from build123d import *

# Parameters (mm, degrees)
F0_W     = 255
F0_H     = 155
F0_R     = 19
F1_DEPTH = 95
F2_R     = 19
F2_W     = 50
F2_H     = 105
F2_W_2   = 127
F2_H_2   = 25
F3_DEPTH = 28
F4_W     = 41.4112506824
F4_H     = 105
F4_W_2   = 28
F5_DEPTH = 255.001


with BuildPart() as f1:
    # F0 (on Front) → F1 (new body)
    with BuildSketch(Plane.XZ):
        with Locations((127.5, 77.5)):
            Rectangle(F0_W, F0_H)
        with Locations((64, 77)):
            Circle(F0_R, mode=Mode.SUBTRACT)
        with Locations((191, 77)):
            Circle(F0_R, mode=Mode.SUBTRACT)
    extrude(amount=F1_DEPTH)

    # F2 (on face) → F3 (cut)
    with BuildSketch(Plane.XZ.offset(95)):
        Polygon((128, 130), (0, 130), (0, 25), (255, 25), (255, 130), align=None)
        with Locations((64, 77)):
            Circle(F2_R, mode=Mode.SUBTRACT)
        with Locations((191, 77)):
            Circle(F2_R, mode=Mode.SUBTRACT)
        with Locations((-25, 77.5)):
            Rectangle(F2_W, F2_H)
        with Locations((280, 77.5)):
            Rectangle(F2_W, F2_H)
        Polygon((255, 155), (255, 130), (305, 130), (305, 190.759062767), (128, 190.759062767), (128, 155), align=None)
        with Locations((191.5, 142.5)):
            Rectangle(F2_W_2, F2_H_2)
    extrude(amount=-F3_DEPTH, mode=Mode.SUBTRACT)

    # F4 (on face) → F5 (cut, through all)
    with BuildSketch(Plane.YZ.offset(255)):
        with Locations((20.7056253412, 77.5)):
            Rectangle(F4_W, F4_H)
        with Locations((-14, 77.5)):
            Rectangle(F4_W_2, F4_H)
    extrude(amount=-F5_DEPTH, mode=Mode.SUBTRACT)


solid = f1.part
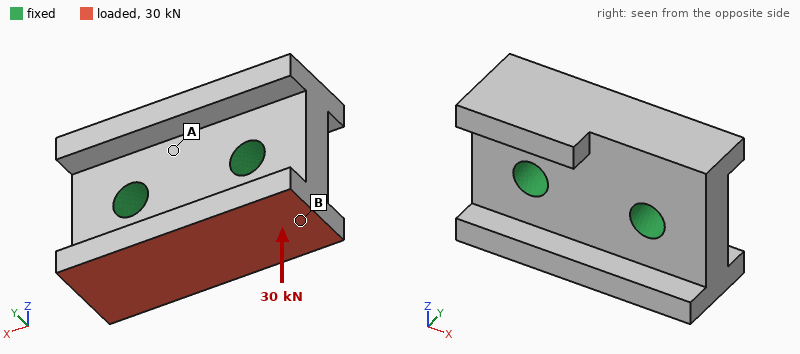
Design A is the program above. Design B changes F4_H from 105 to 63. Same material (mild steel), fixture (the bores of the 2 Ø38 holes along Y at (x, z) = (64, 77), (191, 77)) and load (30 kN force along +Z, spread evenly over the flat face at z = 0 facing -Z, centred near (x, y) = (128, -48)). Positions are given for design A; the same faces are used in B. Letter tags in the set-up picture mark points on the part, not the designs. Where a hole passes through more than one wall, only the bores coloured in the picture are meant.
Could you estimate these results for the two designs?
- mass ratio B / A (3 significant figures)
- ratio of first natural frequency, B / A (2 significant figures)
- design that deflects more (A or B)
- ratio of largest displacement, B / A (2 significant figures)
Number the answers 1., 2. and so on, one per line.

1. 1.14
2. 0.97
3. B
4. 1.1
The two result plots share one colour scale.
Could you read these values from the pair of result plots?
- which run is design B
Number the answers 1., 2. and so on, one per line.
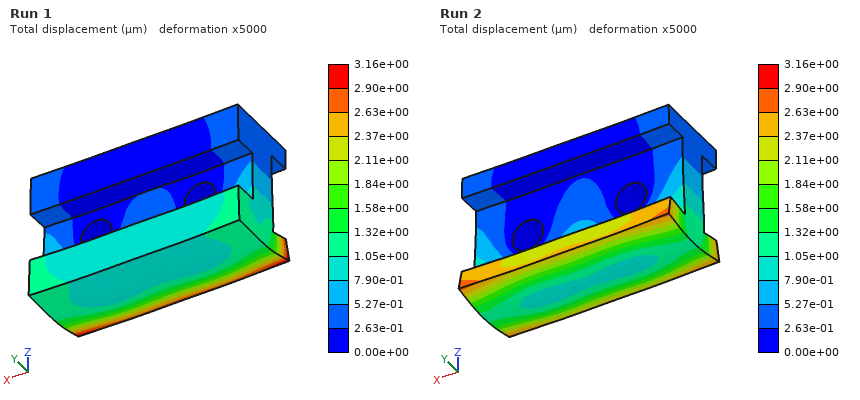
1. Run 1
